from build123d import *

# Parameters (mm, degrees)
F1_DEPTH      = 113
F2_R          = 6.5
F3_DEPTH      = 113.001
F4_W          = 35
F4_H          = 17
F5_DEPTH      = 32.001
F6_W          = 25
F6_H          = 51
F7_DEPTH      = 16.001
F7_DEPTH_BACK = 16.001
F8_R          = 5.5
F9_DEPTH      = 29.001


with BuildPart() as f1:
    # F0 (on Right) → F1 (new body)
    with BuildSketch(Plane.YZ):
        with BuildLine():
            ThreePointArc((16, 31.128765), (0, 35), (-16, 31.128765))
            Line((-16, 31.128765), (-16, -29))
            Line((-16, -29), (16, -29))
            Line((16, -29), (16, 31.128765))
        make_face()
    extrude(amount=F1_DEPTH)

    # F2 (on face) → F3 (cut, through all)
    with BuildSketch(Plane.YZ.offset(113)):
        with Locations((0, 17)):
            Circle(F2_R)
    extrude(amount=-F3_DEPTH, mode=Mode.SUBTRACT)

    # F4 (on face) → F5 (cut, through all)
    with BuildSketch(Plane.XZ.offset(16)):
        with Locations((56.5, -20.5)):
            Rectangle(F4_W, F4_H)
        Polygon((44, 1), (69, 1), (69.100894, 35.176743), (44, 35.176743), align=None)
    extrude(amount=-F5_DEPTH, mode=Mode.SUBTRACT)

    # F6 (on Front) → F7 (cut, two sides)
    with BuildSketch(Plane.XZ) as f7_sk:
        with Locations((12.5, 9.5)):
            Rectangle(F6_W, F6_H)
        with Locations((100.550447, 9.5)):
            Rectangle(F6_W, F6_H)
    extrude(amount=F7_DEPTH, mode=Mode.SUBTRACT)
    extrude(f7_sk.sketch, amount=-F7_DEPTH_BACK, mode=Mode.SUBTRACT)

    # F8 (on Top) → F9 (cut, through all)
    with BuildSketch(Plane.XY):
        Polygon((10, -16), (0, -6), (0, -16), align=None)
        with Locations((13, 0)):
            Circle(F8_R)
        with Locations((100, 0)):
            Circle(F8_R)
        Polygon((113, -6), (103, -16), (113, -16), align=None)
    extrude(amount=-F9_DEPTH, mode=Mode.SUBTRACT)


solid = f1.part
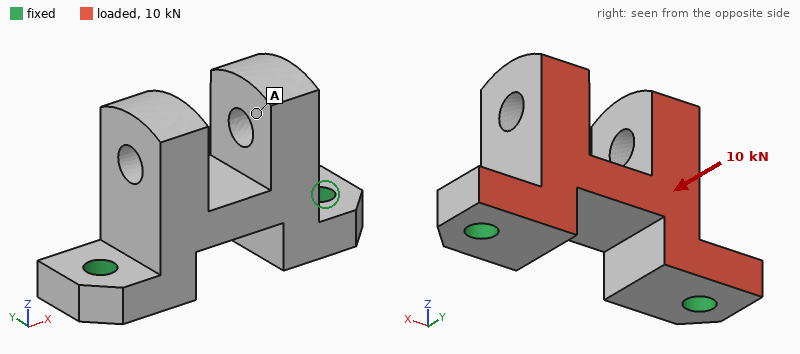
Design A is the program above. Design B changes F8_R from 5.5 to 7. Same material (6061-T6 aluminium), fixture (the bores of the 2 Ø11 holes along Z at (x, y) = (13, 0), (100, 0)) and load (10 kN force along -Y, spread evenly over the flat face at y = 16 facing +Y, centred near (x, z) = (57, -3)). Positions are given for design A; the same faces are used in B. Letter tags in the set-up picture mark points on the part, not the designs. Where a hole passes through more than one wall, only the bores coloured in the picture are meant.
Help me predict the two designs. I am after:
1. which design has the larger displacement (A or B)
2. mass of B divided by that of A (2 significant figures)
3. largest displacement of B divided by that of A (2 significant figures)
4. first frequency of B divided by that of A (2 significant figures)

A
0.98
0.83
1.1
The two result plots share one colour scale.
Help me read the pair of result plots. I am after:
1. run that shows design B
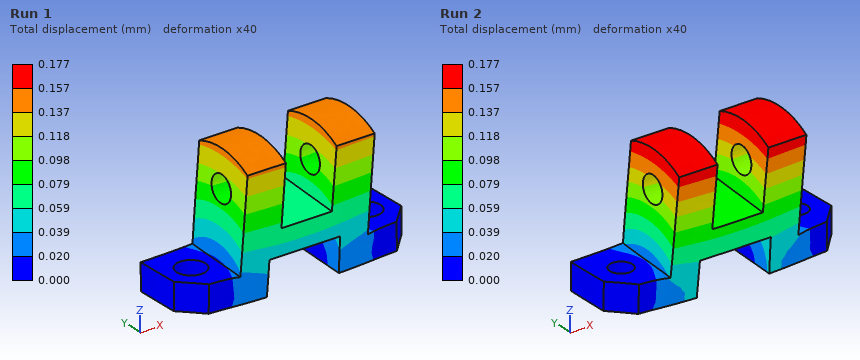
Run 1
